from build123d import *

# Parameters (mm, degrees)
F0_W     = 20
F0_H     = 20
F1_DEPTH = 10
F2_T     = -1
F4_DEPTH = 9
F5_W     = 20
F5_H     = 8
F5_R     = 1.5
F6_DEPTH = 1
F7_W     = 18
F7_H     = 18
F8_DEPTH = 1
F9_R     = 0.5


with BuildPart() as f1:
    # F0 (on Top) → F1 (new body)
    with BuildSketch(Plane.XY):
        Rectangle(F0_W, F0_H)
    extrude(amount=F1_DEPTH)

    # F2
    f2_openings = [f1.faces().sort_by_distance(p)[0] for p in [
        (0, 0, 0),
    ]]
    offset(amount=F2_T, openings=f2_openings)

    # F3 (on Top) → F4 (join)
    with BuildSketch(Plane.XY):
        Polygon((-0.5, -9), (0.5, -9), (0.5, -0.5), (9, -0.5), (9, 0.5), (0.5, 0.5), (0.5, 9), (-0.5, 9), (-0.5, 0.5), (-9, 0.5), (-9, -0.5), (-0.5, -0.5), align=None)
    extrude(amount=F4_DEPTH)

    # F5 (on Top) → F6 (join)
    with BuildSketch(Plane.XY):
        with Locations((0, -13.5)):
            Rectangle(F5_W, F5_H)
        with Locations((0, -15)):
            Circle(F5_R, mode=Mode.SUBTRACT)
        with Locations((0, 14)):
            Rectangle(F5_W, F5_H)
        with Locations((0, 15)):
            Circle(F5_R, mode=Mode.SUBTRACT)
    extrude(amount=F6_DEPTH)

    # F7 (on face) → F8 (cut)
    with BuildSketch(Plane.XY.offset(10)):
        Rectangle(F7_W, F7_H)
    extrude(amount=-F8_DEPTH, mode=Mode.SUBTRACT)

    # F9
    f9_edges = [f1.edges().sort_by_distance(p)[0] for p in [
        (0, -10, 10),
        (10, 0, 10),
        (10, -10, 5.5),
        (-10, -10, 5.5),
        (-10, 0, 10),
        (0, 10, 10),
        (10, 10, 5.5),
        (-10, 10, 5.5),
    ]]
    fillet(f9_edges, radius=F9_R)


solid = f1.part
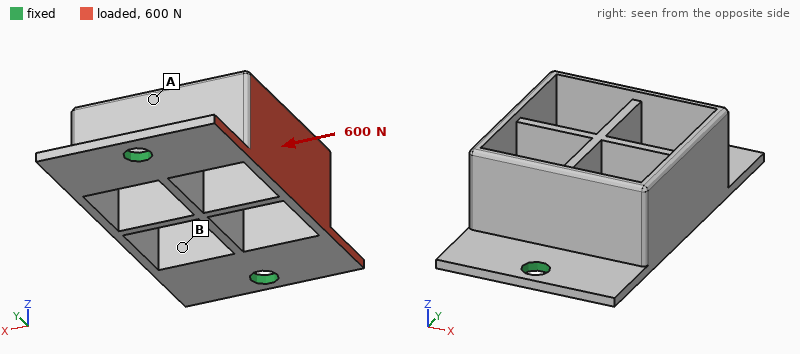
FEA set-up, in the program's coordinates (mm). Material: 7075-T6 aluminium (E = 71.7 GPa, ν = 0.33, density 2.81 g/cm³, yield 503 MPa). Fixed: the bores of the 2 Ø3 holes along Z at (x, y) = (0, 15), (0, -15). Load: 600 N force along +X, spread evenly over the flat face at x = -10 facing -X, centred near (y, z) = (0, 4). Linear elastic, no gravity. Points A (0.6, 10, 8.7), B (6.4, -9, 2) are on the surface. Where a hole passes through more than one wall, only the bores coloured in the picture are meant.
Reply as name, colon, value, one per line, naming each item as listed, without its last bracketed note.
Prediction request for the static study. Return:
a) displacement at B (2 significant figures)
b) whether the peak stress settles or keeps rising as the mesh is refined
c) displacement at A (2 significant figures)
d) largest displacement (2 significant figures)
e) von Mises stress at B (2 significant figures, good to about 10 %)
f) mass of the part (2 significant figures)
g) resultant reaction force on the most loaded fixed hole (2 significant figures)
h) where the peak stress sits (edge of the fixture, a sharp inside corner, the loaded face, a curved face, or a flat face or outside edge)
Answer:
displacement at B: 0.17 mm
whether the peak stress settles or keeps rising as the mesh is refined: keeps rising
displacement at A: 0.21 mm
largest displacement: 0.40 mm
von Mises stress at B: 79 MPa
mass of the part: 3.8 g
resultant reaction force on the most loaded fixed hole: 300 N
where the peak stress sits: edge of the fixture
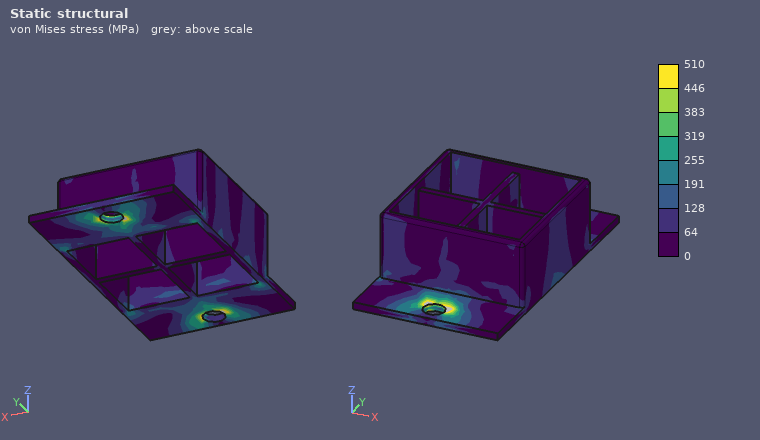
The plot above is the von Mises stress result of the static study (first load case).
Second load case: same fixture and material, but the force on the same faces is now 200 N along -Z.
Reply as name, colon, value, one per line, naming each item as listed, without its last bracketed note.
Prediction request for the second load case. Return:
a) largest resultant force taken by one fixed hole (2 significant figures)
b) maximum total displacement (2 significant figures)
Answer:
largest resultant force taken by one fixed hole: 130 N
maximum total displacement: 0.30 mm
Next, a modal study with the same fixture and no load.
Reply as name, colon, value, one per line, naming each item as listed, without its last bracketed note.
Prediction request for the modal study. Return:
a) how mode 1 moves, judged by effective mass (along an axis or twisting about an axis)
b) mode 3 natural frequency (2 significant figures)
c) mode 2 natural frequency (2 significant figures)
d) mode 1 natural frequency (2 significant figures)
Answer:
how mode 1 moves, judged by effective mass: along X
mode 3 natural frequency: 9000 Hz
mode 2 natural frequency: 9000 Hz
mode 1 natural frequency: 3200 Hz
